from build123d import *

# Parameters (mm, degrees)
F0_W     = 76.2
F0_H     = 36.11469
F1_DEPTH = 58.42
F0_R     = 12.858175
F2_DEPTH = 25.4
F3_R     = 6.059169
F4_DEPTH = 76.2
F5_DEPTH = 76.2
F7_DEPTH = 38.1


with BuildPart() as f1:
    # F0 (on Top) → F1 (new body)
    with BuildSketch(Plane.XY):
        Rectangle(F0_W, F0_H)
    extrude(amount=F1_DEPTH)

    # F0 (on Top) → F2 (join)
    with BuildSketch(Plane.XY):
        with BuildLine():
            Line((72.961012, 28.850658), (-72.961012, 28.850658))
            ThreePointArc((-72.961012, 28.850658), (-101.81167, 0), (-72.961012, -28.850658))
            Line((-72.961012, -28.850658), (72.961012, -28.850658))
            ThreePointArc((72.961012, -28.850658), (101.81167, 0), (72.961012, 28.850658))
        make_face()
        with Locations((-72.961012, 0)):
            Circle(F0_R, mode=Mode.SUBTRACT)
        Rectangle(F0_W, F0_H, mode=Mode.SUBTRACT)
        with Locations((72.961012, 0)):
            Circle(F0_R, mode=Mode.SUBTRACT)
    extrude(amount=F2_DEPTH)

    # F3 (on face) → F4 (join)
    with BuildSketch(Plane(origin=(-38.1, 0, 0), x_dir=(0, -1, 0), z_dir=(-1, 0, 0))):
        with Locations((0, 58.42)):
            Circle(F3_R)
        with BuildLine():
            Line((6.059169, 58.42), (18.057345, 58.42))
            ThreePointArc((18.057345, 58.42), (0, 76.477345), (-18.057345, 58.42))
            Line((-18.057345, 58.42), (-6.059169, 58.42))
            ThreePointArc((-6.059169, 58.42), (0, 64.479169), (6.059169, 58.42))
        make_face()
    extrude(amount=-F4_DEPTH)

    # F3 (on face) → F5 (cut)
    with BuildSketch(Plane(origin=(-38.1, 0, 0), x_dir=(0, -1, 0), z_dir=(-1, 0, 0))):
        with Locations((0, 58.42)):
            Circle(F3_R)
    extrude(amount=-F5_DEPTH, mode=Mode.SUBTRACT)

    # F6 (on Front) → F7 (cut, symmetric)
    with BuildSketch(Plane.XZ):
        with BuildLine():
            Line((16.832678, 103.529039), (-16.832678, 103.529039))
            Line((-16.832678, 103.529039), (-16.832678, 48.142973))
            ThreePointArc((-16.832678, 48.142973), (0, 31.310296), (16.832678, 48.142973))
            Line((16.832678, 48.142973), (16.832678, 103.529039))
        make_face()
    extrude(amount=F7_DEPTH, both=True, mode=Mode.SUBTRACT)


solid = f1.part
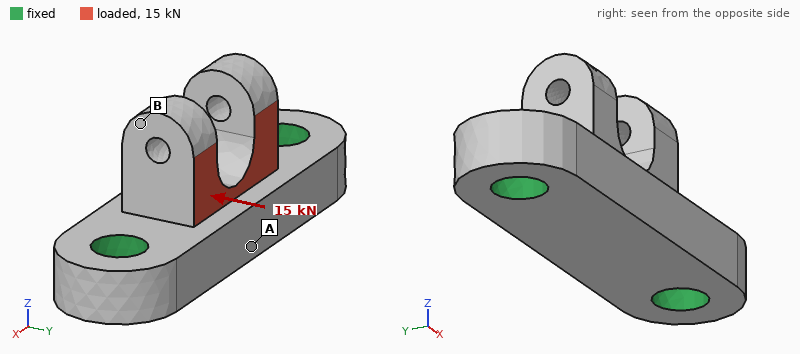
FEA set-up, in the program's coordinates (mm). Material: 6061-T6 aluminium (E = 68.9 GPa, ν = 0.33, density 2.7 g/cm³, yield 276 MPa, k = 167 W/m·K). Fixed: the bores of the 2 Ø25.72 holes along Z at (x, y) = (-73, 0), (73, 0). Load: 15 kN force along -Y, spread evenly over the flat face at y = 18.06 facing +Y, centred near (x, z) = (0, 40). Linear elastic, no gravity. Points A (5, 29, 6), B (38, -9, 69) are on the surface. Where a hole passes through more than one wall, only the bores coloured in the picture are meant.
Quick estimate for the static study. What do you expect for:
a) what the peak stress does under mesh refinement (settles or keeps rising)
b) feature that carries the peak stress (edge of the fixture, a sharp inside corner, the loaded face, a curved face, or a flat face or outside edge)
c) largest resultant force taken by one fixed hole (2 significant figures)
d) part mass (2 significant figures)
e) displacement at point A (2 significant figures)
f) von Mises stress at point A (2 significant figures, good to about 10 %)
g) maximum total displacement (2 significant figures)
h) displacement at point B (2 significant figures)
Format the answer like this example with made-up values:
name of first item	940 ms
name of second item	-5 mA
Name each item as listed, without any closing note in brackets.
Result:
what the peak stress does under mesh refinement	keeps rising
feature that carries the peak stress	edge of the fixture
largest resultant force taken by one fixed hole	7.5 kN
part mass	900 g
displacement at point A	32 µm
von Mises stress at point A	13 MPa
maximum total displacement	94 µm
displacement at point B	84 µm
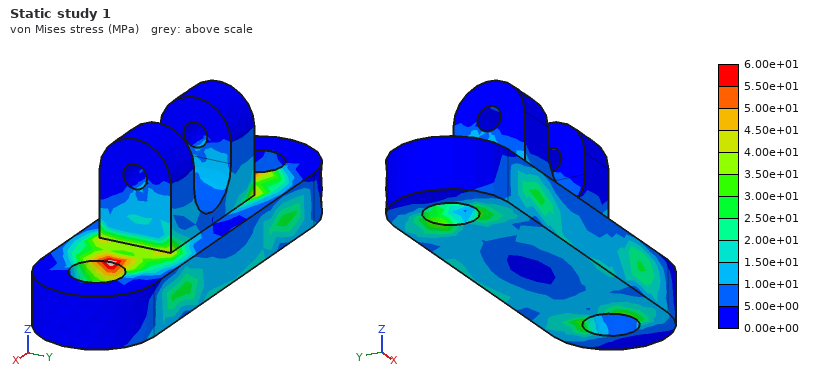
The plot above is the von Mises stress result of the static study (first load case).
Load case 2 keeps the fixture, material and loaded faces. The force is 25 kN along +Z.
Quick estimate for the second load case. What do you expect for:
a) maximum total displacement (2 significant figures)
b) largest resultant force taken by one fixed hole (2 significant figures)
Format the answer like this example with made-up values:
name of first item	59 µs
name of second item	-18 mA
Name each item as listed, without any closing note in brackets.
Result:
maximum total displacement	0.11 mm
largest resultant force taken by one fixed hole	13 kN
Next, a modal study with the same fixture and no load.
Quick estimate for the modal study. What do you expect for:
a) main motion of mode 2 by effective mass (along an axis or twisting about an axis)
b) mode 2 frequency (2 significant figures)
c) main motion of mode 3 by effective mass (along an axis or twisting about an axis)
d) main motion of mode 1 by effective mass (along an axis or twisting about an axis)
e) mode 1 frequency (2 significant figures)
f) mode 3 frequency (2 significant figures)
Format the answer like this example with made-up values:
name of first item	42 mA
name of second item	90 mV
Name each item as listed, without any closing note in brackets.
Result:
main motion of mode 2 by effective mass	along Z
mode 2 frequency	5300 Hz
main motion of mode 3 by effective mass	along X
main motion of mode 1 by effective mass	along Y
mode 1 frequency	4300 Hz
mode 3 frequency	7100 Hz
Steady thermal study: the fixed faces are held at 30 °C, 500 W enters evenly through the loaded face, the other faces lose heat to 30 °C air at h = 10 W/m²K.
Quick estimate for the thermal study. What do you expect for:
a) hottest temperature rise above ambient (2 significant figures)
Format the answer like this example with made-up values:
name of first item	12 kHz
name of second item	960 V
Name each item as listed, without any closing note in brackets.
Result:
hottest temperature rise above ambient	83 K
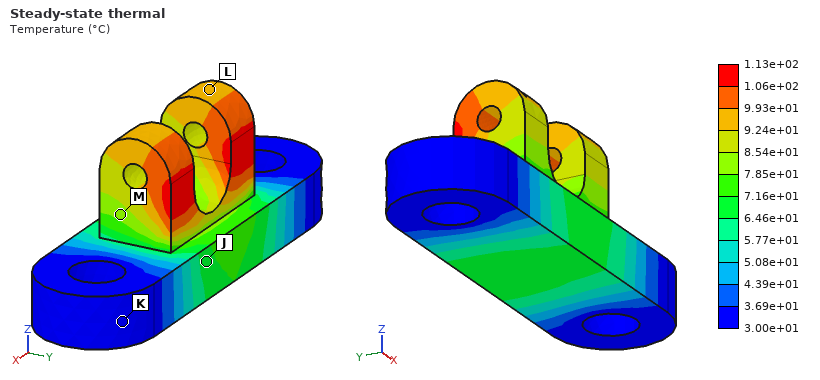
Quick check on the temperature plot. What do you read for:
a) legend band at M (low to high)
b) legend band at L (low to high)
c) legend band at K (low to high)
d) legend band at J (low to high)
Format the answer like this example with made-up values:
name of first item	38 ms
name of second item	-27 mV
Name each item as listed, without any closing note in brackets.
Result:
legend band at M	7.85e+01 to 8.54e+01 °C
legend band at L	9.24e+01 to 9.93e+01 °C
legend band at K	3.00e+01 to 3.69e+01 °C
legend band at J	6.46e+01 to 7.16e+01 °C
